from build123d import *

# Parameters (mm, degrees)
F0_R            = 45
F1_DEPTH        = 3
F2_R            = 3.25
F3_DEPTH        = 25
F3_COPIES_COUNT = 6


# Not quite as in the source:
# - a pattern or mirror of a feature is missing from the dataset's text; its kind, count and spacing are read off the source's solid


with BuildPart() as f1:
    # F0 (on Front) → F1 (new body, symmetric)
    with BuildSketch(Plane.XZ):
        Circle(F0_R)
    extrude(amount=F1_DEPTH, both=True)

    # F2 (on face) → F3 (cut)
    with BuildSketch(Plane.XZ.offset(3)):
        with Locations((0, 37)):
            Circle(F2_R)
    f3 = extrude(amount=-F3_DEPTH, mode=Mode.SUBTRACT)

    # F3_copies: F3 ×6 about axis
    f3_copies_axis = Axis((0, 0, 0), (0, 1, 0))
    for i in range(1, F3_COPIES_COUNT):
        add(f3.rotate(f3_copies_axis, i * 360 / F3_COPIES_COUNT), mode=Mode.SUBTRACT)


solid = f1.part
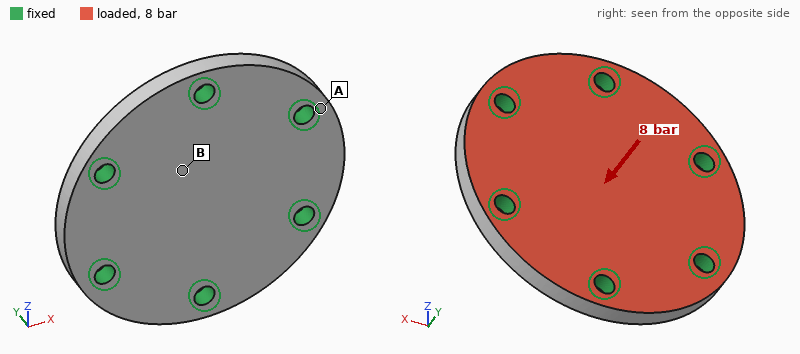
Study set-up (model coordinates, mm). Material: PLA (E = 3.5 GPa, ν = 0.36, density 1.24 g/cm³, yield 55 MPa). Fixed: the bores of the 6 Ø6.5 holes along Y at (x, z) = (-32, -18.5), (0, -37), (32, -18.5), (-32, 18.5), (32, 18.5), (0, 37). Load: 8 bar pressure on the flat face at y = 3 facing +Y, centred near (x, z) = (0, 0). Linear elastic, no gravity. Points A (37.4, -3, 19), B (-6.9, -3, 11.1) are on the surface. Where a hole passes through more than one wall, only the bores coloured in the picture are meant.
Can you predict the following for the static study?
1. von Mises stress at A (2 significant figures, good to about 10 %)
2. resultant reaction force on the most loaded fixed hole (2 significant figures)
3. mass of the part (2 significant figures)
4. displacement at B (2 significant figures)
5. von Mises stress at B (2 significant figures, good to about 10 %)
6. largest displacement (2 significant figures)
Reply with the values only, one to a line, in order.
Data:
5.5 MPa
820 N
46 g
0.32 mm
12 MPa
0.39 mm
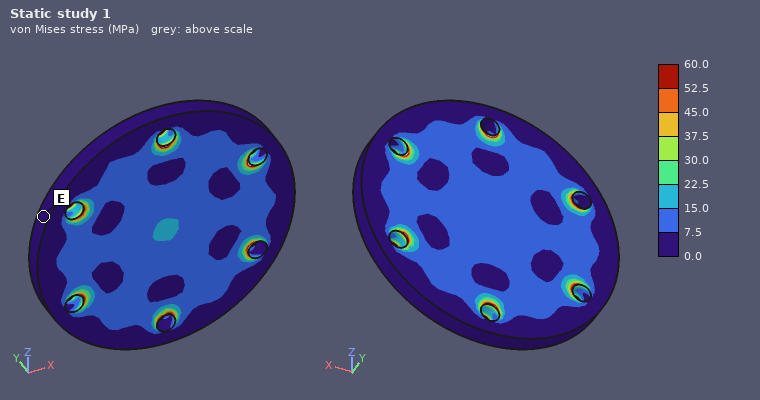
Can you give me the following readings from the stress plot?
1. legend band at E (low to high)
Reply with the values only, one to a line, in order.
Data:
0.0 to 7.5 MPa
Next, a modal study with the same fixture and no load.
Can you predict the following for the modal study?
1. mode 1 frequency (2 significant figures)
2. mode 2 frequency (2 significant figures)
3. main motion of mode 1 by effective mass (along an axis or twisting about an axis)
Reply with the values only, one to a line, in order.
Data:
3200 Hz
6100 Hz
along Y
